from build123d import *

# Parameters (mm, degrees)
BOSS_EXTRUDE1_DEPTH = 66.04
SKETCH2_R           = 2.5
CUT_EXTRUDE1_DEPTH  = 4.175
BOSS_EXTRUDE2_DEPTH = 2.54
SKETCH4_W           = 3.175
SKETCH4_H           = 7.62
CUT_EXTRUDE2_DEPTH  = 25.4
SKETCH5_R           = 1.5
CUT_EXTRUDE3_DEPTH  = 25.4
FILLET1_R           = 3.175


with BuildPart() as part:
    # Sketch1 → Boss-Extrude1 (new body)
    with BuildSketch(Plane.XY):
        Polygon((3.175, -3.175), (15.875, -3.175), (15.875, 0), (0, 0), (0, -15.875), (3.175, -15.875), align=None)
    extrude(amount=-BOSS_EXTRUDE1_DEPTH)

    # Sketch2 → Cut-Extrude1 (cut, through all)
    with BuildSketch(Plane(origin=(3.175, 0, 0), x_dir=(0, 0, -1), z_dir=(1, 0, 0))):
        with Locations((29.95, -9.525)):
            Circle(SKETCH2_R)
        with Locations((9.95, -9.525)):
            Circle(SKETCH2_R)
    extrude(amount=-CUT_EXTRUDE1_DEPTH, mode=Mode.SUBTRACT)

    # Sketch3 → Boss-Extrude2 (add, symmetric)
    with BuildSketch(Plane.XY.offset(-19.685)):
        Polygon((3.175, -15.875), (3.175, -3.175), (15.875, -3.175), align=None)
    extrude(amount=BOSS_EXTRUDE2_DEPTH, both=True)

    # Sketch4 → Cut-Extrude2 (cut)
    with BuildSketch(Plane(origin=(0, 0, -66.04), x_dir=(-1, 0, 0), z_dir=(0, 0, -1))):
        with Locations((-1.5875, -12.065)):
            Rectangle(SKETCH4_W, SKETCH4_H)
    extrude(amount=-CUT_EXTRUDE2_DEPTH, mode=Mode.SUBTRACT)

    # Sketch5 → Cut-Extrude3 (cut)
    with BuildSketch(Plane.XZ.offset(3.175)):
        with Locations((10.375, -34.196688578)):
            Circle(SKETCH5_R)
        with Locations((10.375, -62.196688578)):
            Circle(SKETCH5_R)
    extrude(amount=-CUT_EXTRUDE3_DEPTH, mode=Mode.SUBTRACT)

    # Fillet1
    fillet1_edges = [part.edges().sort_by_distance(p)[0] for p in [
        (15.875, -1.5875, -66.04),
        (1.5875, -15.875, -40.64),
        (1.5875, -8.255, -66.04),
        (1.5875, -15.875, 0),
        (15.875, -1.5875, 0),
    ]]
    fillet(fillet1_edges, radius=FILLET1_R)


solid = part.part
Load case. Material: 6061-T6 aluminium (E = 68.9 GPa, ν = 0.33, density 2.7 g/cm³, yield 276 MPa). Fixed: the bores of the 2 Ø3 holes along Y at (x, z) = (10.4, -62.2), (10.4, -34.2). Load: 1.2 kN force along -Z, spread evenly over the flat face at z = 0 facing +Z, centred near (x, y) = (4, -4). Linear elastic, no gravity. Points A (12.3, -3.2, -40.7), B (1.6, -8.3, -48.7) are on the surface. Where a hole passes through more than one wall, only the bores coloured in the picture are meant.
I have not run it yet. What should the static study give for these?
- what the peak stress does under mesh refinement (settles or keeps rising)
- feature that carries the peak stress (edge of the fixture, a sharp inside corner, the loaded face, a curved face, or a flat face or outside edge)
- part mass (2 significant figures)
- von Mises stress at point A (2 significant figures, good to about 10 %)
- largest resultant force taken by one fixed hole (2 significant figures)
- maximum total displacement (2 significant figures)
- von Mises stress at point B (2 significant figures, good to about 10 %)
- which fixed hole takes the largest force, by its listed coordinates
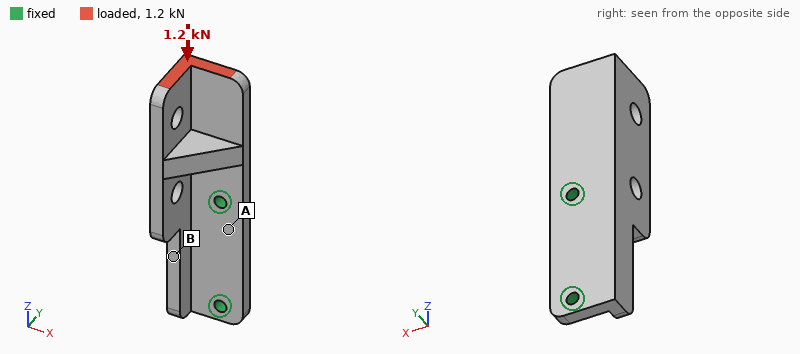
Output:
keeps rising
edge of the fixture
15 g
9.2 MPa
850 N
49 µm
23 MPa
(10.4, -34.2)
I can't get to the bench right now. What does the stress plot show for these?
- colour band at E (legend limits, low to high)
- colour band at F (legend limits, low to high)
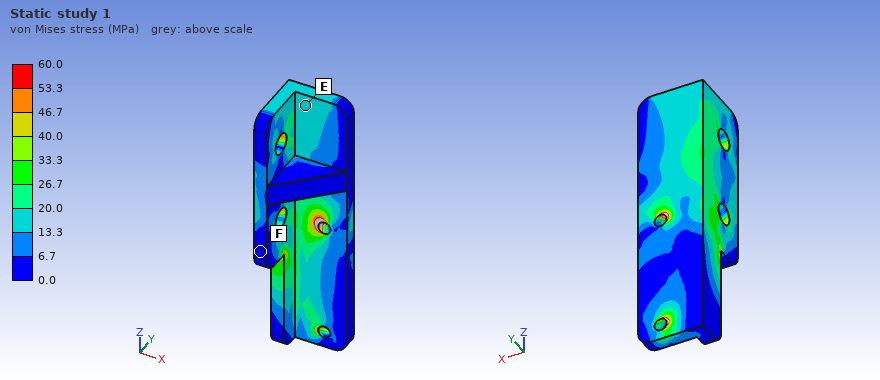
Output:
13.3 to 20.0 MPa
0.0 to 6.7 MPa
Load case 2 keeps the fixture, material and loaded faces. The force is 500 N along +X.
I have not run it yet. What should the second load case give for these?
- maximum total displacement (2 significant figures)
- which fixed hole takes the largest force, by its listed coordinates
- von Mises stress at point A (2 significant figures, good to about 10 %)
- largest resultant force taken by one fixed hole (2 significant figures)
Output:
0.24 mm
(10.4, -34.2)
24 MPa
1.1 kN
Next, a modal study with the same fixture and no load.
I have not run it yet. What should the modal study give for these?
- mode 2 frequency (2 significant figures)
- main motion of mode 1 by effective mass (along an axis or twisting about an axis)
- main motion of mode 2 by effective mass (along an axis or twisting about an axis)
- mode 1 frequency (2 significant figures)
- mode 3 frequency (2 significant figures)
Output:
5300 Hz
along Y
along X
3000 Hz
6900 Hz
